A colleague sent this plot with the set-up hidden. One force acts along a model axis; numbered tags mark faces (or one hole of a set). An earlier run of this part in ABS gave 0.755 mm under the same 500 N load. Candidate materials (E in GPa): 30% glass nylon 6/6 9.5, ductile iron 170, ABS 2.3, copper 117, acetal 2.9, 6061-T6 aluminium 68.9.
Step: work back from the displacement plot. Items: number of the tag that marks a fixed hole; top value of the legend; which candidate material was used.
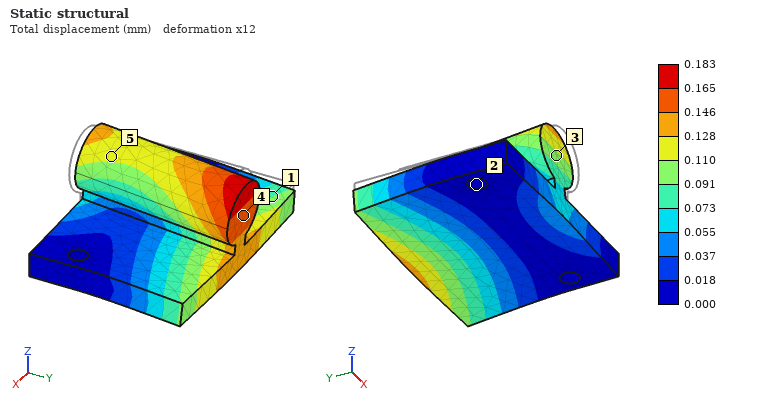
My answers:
2
0.183 mm
30% glass nylon 6/6
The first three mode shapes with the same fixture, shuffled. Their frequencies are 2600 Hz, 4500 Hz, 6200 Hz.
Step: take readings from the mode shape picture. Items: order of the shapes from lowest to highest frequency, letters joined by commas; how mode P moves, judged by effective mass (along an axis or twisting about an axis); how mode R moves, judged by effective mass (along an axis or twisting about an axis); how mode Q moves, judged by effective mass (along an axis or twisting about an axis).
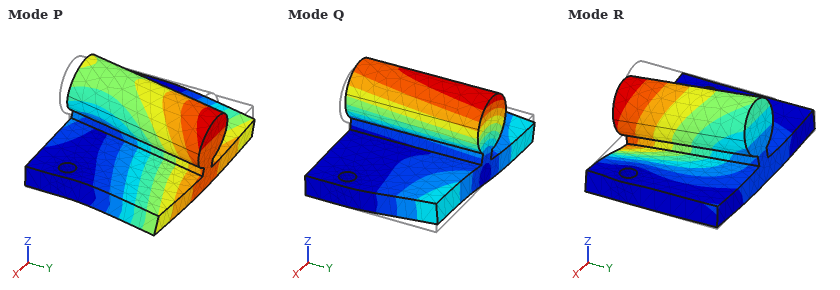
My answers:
P, Q, R
along Z
along Z
along X
